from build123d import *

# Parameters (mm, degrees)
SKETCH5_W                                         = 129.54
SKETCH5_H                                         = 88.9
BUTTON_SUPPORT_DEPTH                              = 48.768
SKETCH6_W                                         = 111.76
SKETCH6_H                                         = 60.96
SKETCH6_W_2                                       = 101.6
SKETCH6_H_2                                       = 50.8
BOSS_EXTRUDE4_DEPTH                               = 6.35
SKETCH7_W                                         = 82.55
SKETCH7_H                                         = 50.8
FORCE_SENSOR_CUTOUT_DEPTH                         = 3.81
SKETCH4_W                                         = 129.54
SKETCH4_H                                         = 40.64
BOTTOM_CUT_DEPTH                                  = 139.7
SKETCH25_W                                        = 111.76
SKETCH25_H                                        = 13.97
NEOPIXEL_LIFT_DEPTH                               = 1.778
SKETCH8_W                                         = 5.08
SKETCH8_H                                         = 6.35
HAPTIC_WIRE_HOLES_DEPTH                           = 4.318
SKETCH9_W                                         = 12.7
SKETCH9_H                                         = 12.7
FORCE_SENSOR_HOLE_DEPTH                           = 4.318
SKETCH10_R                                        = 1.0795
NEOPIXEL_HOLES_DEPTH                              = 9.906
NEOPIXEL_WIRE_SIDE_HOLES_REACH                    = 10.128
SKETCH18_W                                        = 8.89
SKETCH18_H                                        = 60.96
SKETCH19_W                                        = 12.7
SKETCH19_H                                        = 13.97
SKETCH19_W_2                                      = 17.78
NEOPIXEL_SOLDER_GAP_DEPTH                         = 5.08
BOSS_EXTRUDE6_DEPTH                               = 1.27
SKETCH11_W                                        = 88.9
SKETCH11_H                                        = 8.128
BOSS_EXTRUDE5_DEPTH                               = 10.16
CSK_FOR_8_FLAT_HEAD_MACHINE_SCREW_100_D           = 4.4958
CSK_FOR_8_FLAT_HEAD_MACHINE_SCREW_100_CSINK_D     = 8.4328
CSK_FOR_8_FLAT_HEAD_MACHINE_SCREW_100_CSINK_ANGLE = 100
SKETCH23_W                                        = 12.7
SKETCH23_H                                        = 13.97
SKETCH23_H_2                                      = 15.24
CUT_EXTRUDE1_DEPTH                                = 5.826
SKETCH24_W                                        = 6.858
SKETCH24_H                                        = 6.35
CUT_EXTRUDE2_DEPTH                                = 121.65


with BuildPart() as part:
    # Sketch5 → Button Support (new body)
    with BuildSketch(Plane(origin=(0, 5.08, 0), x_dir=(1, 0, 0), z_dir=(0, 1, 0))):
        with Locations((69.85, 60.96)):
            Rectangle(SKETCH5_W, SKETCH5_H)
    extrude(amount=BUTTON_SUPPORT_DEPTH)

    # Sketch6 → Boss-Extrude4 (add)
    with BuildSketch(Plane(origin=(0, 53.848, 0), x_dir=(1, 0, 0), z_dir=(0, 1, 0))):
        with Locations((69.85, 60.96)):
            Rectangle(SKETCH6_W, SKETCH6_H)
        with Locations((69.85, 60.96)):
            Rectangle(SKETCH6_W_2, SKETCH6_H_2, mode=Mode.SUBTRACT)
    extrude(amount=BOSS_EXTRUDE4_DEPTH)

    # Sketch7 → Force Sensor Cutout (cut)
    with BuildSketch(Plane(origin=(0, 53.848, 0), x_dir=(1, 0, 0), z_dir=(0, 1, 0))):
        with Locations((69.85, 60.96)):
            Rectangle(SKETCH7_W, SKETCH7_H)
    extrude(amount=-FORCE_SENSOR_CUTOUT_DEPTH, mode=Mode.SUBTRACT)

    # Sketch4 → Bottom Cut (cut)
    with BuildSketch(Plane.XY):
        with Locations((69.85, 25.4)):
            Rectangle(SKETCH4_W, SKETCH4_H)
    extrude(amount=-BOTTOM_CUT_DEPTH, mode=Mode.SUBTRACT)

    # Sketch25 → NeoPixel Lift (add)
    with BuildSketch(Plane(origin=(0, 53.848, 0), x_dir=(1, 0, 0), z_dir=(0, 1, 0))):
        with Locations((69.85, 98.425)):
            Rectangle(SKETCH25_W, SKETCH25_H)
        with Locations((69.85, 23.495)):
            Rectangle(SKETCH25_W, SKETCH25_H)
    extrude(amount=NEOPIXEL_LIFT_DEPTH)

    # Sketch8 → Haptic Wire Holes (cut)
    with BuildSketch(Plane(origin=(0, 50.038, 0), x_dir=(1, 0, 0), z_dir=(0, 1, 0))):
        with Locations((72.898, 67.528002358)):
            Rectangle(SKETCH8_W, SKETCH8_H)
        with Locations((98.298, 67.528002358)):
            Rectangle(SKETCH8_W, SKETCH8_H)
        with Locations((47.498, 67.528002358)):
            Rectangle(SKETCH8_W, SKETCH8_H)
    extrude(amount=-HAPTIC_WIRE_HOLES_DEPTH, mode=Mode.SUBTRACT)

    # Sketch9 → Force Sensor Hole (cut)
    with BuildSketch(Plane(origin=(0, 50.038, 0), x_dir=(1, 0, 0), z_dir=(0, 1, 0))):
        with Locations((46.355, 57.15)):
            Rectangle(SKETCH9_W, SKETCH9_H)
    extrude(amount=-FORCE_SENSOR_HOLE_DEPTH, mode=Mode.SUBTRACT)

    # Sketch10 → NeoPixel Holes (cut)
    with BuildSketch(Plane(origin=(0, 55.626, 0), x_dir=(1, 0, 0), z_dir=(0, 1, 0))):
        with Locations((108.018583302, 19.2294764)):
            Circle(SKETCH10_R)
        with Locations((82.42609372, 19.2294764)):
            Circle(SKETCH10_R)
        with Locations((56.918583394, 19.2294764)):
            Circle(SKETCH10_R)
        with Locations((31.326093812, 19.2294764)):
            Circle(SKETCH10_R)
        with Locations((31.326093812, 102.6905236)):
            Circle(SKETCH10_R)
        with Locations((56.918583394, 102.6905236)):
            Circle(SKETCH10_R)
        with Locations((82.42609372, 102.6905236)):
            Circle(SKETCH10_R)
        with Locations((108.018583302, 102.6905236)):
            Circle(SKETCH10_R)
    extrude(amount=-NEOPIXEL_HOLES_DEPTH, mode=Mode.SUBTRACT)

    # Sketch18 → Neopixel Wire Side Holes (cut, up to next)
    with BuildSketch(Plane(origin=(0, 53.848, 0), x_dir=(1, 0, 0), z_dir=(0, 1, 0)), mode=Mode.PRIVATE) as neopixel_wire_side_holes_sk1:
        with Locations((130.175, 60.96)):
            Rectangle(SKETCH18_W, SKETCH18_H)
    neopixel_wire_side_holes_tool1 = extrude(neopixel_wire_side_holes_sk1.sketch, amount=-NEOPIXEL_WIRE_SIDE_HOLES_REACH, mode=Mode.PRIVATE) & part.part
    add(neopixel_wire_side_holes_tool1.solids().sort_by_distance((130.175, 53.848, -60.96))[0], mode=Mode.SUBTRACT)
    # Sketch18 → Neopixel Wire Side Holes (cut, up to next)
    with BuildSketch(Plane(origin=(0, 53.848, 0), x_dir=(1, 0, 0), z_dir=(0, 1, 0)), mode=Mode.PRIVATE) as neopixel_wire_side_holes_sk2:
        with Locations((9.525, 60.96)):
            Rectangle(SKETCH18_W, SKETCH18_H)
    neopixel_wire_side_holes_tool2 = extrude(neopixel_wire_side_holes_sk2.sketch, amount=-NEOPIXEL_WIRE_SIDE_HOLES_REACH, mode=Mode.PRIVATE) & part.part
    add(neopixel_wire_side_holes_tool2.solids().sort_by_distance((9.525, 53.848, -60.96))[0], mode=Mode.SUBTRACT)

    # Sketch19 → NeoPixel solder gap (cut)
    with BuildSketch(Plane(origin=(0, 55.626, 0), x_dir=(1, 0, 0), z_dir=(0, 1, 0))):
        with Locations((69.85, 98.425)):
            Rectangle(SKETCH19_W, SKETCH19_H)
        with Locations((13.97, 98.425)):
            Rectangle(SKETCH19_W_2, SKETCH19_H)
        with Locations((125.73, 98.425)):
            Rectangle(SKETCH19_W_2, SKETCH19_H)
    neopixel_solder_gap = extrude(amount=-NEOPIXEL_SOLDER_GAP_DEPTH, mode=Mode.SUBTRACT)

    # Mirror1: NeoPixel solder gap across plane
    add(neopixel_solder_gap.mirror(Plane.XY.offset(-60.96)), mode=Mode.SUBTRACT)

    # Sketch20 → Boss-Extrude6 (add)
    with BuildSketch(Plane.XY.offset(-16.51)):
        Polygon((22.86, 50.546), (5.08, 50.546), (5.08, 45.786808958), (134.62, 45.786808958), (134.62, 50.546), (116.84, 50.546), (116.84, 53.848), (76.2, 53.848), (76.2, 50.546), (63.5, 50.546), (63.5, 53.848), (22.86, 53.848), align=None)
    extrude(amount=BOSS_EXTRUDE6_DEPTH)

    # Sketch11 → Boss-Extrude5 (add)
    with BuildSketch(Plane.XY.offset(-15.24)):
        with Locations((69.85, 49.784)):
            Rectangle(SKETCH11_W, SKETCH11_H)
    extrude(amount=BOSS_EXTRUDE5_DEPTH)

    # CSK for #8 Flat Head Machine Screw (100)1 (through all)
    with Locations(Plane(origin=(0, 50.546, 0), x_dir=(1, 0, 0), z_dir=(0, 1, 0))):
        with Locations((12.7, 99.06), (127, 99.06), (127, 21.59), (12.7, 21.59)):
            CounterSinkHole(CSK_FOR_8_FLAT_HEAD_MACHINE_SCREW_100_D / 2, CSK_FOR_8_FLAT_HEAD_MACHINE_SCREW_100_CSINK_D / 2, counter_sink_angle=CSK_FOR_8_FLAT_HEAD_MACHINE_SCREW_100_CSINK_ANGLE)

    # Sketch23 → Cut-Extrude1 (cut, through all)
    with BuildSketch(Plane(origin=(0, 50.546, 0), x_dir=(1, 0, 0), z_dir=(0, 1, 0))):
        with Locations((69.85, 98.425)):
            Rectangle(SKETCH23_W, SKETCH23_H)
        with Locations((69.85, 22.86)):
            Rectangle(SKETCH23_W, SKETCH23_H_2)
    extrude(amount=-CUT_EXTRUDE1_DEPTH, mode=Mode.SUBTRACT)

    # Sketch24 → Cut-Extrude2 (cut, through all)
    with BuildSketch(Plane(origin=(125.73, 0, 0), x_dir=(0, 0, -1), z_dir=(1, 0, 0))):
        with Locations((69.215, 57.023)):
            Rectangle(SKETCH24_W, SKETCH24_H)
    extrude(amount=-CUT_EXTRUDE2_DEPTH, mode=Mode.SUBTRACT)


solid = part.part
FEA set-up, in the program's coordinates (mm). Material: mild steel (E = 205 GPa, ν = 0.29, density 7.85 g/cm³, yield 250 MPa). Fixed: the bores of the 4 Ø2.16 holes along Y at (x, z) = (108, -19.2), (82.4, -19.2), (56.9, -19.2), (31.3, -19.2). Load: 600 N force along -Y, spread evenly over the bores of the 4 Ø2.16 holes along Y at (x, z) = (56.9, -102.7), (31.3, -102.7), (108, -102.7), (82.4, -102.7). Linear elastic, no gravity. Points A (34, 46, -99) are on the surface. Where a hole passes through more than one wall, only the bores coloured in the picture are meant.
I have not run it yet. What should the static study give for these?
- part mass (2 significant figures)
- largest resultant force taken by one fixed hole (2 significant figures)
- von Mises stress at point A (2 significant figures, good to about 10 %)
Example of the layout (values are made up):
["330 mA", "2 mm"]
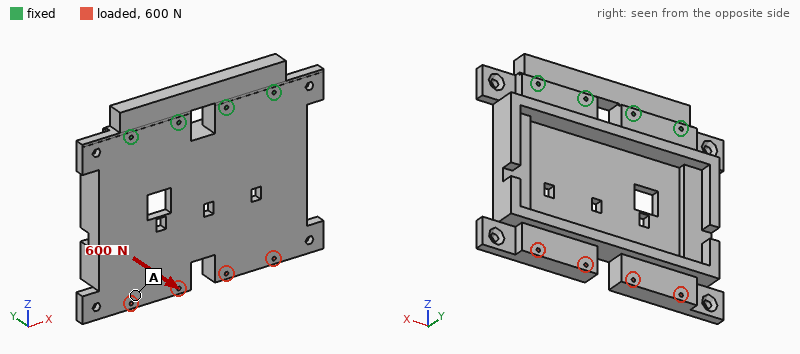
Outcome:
["650 g", "570 N", "6.7 MPa"]
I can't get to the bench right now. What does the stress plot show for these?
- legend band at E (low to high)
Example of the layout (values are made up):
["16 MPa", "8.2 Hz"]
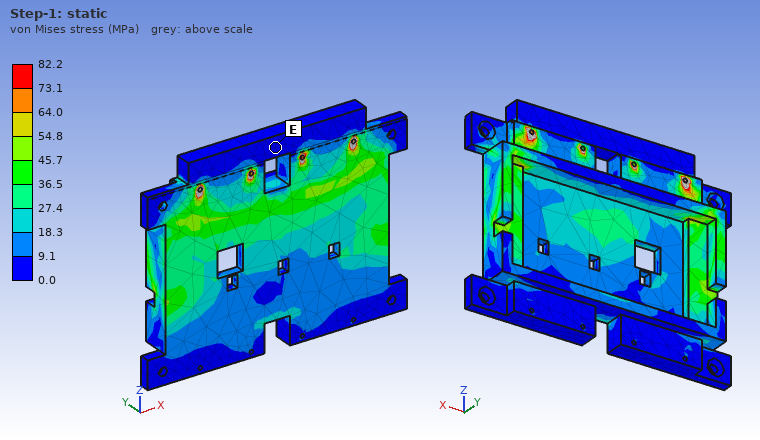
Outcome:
["0.0 to 9.1 MPa"]
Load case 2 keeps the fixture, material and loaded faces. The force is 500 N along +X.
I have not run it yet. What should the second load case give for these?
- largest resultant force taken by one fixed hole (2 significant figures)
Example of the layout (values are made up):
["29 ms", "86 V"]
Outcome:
["570 N"]
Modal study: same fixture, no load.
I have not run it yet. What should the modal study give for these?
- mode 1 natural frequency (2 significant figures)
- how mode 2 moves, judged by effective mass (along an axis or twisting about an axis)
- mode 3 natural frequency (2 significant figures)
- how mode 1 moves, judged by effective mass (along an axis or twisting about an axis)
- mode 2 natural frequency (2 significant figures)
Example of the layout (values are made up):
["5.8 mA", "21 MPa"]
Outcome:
["720 Hz", "twisting about Z", "4100 Hz", "along Y", "1300 Hz"]
